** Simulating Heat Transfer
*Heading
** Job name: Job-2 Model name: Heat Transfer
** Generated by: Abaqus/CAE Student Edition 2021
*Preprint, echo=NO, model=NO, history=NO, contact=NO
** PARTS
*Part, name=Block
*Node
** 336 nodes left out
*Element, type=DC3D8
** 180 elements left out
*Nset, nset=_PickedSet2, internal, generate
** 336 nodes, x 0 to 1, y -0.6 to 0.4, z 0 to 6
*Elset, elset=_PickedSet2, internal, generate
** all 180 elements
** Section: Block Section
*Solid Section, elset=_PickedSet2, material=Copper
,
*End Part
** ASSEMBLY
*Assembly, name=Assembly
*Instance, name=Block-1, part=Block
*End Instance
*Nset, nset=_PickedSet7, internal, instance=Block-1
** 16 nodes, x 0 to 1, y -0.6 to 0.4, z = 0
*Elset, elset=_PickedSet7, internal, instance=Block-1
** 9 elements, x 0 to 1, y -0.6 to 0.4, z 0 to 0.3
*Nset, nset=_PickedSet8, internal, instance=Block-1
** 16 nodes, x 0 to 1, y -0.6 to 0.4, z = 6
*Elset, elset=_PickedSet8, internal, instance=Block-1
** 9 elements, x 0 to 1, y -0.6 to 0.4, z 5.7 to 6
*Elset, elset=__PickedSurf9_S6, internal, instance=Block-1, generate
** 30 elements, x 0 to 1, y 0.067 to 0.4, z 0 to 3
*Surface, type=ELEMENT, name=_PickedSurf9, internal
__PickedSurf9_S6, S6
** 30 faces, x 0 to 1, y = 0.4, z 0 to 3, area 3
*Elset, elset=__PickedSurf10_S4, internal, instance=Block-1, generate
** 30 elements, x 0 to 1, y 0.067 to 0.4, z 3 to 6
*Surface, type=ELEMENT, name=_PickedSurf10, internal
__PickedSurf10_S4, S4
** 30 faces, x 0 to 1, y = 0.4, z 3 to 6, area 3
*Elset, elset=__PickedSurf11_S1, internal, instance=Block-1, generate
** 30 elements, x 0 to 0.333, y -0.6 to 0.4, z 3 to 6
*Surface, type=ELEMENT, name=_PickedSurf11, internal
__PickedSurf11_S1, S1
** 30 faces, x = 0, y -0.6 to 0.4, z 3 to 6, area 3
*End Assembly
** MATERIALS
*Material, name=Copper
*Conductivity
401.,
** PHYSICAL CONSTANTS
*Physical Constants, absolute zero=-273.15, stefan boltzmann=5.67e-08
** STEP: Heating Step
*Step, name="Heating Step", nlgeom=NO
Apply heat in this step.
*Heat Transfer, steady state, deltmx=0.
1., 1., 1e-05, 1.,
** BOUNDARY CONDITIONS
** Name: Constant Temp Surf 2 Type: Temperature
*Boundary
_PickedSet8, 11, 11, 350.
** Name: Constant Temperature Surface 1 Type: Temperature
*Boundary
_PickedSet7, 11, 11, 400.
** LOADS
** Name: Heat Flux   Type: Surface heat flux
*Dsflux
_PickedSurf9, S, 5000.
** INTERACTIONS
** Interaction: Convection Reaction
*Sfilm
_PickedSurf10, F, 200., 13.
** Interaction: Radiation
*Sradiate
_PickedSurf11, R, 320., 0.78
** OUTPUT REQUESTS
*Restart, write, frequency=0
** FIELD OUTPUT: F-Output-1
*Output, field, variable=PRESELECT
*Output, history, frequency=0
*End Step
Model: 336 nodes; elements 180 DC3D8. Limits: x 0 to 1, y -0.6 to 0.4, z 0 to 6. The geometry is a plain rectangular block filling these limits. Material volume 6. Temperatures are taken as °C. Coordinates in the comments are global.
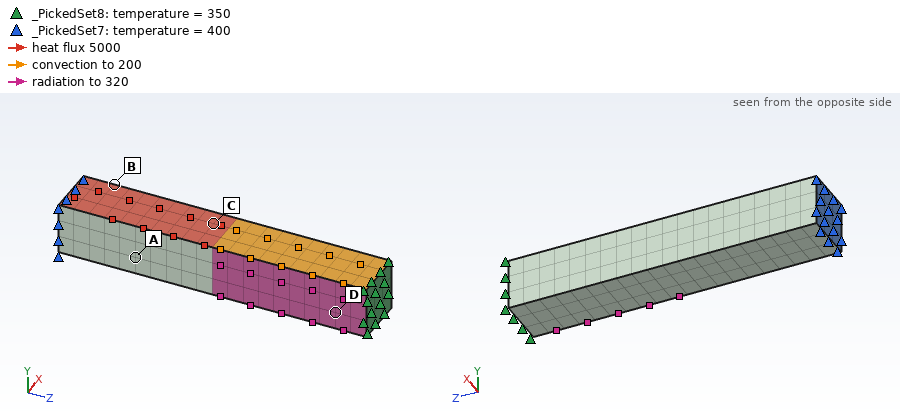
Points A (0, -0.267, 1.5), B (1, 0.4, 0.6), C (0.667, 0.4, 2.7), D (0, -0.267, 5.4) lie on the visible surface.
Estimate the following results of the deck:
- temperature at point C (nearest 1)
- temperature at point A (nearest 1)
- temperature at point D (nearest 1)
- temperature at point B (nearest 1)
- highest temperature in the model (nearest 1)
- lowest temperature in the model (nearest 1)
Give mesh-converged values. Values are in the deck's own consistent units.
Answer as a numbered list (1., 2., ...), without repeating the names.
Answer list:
1. 392 °C
2. 403 °C
3. 350 °C
4. 409 °C
5. 410 °C
6. 348 °C
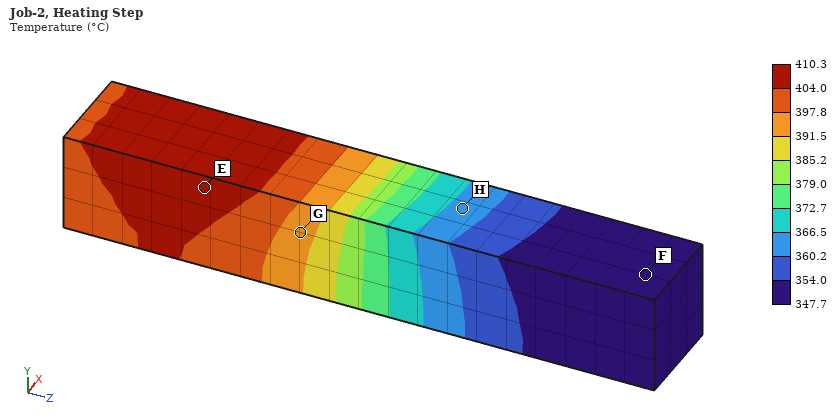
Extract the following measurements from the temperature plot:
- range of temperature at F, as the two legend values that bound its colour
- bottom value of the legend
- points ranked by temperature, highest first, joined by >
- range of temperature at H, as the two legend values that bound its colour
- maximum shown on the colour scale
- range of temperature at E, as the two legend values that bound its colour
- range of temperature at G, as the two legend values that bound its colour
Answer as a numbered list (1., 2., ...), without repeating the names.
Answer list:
1. 347.7 to 354.0 °C
2. 347.7 °C
3. E > G > H > F
4. 360.2 to 366.5 °C
5. 410.3 °C
6. 404.0 to 410.3 °C
7. 391.5 to 397.8 °C
